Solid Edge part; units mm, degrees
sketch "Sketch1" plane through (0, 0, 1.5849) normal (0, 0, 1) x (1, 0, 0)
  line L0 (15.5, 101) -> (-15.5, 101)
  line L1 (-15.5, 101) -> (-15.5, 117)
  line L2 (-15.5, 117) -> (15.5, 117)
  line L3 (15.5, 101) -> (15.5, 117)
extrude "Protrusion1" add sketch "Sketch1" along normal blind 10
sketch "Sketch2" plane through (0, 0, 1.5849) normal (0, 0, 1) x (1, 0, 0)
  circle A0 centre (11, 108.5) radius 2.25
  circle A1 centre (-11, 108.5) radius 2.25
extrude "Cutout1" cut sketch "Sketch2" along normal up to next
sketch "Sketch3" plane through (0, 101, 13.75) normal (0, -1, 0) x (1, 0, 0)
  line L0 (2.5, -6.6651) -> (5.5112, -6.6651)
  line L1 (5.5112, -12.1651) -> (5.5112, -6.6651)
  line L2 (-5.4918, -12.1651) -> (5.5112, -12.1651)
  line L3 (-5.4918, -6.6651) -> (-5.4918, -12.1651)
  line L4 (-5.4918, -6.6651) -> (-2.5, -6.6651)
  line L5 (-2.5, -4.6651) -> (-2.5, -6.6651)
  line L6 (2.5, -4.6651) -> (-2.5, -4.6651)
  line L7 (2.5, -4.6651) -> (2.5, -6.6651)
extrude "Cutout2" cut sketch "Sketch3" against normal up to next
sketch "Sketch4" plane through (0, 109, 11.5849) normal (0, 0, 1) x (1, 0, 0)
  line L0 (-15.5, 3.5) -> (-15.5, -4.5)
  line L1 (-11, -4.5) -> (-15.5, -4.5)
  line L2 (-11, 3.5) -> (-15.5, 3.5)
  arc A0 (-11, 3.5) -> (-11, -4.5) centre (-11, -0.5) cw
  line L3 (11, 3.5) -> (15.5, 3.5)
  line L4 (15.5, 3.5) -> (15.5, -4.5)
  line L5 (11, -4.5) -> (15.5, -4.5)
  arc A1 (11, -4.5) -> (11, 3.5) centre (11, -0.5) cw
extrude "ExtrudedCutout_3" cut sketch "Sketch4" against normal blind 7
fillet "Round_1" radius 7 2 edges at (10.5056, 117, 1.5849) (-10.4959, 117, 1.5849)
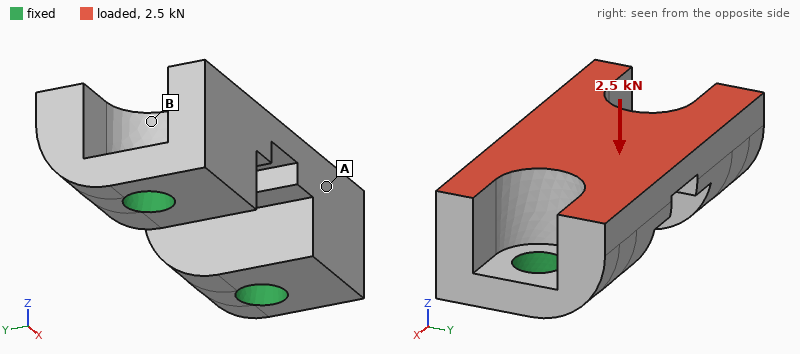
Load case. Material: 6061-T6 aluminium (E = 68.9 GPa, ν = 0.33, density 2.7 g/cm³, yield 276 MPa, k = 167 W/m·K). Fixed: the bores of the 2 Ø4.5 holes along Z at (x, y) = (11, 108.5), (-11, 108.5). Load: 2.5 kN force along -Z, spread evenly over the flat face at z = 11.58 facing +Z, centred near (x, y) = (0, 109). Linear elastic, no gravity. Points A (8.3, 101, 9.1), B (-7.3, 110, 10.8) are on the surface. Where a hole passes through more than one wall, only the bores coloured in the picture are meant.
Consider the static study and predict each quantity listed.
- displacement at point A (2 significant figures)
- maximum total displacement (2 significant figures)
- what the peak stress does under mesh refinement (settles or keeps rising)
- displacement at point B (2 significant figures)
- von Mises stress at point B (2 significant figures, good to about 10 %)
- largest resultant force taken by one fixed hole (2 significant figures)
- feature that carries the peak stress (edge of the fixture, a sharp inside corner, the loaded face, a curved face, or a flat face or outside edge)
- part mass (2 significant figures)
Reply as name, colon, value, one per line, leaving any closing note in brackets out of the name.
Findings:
displacement at point A: 3.9 µm
maximum total displacement: 16 µm
what the peak stress does under mesh refinement: keeps rising
displacement at point B: 7.9 µm
von Mises stress at point B: 31 MPa
largest resultant force taken by one fixed hole: 1.3 kN
feature that carries the peak stress: edge of the fixture
part mass: 7.2 g
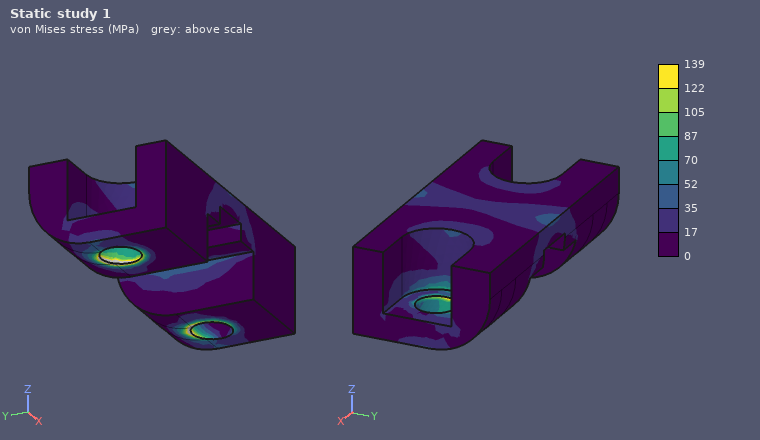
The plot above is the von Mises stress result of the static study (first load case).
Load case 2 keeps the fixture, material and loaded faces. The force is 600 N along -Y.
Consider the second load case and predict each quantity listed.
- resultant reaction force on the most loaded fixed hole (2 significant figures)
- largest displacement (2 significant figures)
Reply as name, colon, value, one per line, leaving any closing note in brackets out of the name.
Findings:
resultant reaction force on the most loaded fixed hole: 300 N
largest displacement: 21 µm
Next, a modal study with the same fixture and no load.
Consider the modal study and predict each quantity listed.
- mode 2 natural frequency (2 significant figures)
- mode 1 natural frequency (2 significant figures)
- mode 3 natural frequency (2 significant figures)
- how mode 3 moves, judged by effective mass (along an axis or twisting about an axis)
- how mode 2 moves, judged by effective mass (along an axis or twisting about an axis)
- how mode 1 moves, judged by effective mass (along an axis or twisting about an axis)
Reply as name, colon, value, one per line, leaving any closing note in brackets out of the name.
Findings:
mode 2 natural frequency: 24 kHz
mode 1 natural frequency: 16 kHz
mode 3 natural frequency: 29 kHz
how mode 3 moves, judged by effective mass: along X
how mode 2 moves, judged by effective mass: twisting about Z
how mode 1 moves, judged by effective mass: along Y
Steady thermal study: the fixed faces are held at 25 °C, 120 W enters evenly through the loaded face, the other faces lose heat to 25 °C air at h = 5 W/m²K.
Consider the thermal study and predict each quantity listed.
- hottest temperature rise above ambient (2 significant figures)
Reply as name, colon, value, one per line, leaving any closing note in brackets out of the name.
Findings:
hottest temperature rise above ambient: 58 K
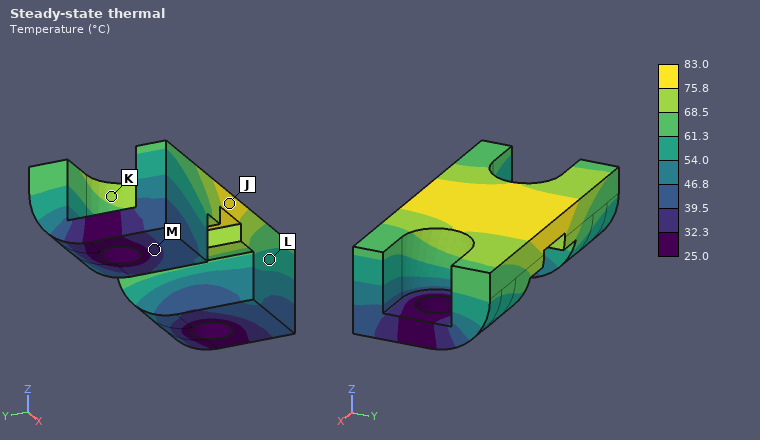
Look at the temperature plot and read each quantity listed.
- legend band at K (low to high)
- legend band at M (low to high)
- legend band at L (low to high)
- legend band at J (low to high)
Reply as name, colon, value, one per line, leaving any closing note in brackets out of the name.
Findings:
legend band at K: 68.5 to 75.8 °C
legend band at M: 32.3 to 39.5 °C
legend band at L: 54.0 to 61.3 °C
legend band at J: 75.8 to 83.0 °C
